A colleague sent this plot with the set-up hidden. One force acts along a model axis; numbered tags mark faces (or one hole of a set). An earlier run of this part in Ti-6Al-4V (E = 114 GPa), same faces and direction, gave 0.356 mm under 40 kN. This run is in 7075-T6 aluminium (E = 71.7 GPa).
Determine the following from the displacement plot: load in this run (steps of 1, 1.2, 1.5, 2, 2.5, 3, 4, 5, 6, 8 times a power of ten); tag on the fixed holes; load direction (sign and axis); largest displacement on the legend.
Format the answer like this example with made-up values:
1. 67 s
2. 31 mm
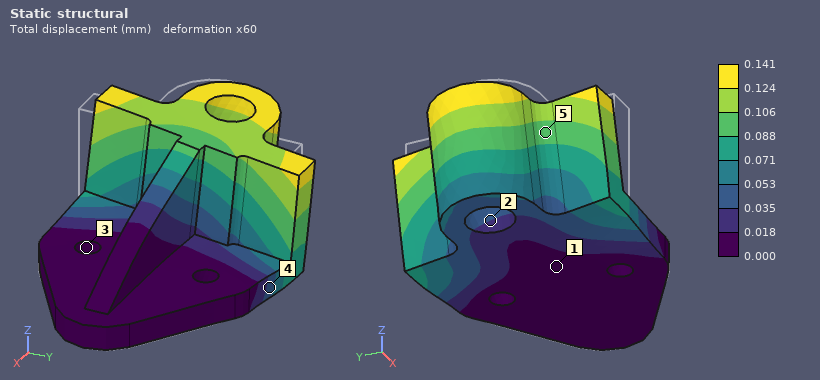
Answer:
1. 10 kN
2. 3
3. +Y
4. 0.141 mm
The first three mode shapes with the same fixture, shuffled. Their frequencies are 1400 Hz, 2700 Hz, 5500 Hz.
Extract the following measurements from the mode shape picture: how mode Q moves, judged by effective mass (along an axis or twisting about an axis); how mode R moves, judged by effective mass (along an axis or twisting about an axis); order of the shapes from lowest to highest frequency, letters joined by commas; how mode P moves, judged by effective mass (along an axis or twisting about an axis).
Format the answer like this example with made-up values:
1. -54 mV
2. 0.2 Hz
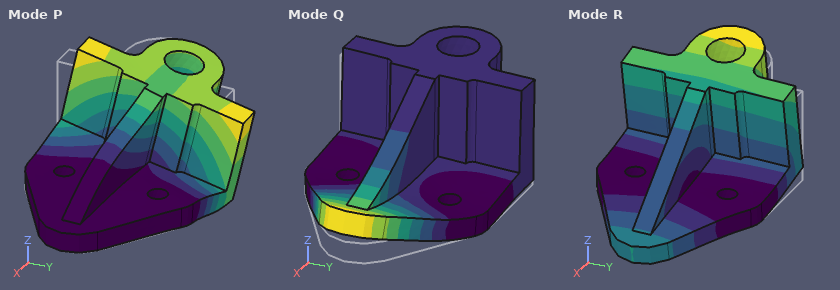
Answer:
1. along Z
2. along Z
3. R, P, Q
4. along Y
